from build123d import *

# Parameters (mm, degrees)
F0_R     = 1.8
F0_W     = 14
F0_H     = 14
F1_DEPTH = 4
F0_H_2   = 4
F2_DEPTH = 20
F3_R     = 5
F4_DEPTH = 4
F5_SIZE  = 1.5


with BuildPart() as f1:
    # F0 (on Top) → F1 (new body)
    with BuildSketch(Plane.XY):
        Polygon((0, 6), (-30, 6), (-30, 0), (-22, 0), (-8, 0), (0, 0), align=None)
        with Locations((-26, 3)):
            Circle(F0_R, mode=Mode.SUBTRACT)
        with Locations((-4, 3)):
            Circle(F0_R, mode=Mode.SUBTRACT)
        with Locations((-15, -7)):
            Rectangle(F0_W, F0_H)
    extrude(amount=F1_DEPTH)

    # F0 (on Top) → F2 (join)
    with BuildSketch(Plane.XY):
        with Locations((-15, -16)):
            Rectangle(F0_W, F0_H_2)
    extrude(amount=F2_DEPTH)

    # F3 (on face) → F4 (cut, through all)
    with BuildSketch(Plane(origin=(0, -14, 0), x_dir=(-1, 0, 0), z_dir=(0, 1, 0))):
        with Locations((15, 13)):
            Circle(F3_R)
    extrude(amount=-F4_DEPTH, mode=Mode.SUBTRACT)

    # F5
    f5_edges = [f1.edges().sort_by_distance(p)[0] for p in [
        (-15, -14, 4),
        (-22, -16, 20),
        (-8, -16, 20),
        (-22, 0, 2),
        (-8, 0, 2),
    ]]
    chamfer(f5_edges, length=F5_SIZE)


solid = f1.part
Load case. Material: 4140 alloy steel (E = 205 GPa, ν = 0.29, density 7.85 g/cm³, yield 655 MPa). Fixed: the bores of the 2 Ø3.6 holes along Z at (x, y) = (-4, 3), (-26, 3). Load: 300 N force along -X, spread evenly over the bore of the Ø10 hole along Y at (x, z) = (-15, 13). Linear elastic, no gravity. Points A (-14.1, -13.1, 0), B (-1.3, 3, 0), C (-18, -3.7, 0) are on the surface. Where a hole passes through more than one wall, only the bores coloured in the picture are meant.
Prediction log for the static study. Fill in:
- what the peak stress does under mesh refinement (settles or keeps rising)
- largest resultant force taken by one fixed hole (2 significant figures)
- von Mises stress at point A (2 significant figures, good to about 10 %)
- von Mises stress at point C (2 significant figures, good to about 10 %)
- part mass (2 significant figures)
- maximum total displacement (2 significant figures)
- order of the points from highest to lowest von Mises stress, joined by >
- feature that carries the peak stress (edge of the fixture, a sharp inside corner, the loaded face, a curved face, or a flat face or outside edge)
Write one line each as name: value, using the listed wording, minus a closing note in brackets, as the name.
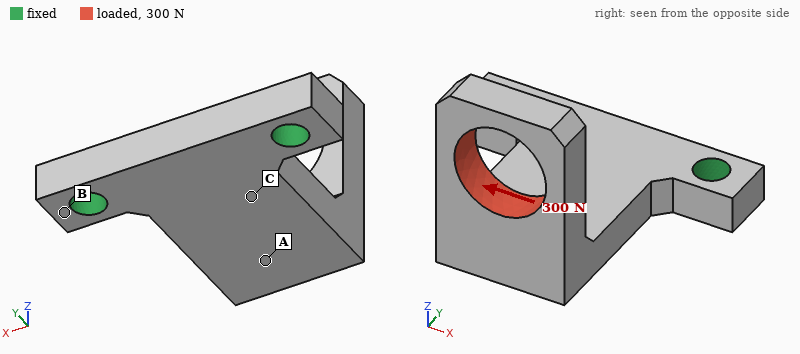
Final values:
what the peak stress does under mesh refinement: keeps rising
largest resultant force taken by one fixed hole: 400 N
von Mises stress at point A: 45 MPa
von Mises stress at point C: 66 MPa
part mass: 18 g
maximum total displacement: 54 µm
order of the points from highest to lowest von Mises stress, joined by >: C > A > B
feature that carries the peak stress: edge of the fixture
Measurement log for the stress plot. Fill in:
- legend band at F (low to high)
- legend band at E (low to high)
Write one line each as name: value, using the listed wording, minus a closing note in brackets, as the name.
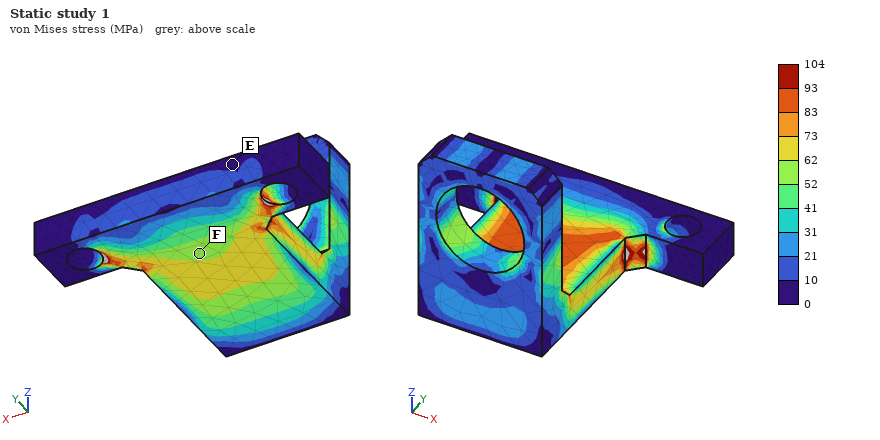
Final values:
legend band at F: 52 to 62 MPa
legend band at E: 0 to 10 MPa
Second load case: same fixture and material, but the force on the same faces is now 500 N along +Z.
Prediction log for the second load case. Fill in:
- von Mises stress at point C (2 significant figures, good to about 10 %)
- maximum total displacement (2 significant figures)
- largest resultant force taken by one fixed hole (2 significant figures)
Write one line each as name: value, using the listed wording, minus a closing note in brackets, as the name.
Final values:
von Mises stress at point C: 160 MPa
maximum total displacement: 0.19 mm
largest resultant force taken by one fixed hole: 250 N
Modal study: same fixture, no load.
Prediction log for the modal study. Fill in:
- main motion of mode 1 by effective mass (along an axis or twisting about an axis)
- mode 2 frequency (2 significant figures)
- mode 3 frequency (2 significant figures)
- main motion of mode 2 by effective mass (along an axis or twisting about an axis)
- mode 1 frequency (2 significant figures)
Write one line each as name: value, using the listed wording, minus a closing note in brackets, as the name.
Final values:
main motion of mode 1 by effective mass: along Z
mode 2 frequency: 6700 Hz
mode 3 frequency: 9500 Hz
main motion of mode 2 by effective mass: along X
mode 1 frequency: 3200 Hz
